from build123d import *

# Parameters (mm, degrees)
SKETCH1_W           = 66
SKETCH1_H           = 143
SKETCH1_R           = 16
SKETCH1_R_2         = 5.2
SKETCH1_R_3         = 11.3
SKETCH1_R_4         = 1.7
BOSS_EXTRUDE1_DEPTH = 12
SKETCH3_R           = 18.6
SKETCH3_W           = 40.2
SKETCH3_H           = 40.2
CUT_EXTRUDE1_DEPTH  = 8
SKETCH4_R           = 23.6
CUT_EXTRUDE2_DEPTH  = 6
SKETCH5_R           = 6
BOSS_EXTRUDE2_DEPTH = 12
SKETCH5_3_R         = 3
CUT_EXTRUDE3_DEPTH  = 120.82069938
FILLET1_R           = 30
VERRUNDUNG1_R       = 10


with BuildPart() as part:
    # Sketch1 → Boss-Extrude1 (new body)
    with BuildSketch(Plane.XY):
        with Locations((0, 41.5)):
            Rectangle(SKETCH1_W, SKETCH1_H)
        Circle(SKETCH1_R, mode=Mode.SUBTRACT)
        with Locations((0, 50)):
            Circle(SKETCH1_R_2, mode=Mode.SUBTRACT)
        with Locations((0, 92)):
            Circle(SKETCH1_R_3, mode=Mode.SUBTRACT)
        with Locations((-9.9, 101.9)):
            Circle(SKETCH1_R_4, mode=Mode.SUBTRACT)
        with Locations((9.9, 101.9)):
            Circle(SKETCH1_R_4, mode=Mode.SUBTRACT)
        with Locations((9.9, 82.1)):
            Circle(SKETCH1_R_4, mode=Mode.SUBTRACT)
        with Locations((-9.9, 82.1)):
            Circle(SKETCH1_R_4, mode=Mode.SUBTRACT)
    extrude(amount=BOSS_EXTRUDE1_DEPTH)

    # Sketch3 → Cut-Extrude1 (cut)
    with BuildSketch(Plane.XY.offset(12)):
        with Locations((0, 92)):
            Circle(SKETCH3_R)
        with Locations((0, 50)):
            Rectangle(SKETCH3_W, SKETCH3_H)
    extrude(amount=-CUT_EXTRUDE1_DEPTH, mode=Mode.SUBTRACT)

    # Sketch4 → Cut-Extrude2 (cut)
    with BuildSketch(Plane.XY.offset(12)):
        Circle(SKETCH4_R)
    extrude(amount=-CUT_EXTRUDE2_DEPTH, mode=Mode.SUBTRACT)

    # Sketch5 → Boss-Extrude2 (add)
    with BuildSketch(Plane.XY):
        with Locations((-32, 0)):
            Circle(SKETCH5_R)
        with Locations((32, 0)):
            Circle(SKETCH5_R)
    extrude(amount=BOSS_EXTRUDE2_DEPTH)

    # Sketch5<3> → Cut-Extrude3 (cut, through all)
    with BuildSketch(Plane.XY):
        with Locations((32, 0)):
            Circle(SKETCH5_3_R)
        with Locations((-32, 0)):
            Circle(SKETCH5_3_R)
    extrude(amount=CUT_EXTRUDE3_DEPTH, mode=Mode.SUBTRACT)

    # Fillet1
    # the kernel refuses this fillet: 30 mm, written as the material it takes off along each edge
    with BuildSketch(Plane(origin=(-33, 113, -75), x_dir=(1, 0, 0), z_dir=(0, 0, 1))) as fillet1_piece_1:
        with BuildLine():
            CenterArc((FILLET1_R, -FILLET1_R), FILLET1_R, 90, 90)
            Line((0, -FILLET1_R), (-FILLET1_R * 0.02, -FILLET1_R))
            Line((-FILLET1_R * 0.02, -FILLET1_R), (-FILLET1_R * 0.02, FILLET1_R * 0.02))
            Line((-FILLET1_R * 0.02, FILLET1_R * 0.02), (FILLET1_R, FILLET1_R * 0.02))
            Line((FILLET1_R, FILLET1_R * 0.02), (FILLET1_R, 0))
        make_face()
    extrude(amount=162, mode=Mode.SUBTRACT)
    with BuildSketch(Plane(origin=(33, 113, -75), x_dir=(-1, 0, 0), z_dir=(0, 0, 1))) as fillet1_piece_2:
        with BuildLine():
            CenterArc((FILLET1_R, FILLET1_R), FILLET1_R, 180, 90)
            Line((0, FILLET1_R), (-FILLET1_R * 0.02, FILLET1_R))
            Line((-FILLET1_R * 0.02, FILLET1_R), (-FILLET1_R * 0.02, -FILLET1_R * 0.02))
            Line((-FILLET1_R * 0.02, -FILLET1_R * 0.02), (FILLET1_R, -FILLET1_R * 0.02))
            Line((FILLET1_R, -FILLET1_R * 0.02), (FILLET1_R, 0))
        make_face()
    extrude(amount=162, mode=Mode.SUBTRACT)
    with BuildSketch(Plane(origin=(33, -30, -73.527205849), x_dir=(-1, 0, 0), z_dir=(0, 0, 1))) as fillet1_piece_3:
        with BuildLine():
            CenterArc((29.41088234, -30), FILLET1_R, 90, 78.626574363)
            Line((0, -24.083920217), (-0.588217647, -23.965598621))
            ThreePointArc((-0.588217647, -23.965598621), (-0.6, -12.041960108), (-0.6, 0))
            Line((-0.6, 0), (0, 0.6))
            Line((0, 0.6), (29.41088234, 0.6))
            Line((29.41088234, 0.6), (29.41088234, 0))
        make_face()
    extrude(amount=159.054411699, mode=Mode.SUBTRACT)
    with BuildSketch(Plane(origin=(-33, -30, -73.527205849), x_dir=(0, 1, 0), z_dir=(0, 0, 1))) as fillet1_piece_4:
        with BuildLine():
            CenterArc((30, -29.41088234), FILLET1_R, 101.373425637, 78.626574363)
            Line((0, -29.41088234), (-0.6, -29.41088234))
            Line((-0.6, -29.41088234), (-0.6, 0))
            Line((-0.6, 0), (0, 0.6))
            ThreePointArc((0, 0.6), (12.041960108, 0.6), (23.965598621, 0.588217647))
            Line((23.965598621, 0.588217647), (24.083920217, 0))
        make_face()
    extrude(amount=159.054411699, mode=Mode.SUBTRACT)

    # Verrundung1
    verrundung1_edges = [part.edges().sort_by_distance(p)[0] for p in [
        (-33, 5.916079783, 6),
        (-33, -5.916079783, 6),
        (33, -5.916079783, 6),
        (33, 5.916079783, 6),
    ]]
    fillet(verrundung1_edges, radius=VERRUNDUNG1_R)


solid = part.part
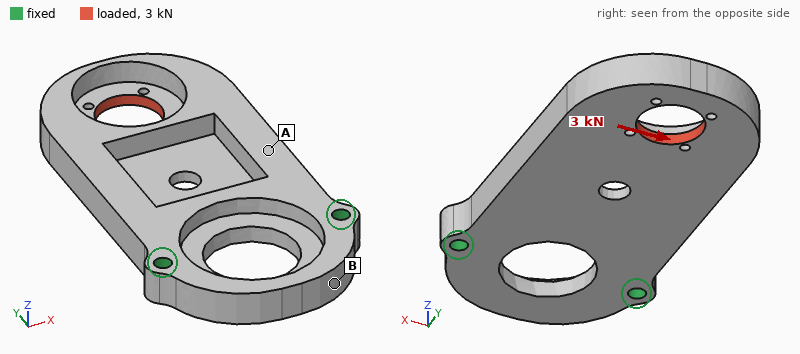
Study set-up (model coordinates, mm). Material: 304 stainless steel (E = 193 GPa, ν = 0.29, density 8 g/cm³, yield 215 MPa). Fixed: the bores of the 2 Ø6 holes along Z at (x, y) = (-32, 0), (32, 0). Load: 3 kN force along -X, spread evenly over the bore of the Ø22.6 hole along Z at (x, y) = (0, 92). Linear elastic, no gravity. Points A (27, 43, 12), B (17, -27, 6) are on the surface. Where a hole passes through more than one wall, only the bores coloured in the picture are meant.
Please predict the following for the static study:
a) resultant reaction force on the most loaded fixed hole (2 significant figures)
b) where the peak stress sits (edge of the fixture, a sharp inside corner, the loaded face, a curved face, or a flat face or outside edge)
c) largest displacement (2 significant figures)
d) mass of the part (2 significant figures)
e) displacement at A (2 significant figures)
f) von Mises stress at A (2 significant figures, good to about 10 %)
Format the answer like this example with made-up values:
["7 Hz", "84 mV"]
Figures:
["4.6 kN", "a curved face", "44 µm", "530 g", "11 µm", "15 MPa"]
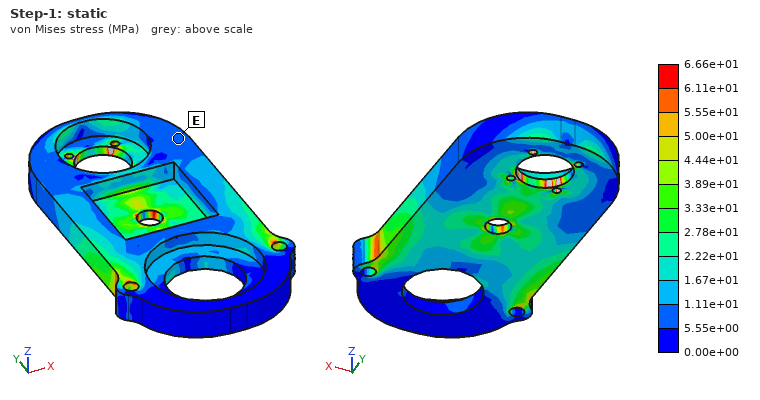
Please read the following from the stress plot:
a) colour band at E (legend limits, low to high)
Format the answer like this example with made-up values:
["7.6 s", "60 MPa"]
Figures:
["5.55e+00 to 1.11e+01 MPa"]
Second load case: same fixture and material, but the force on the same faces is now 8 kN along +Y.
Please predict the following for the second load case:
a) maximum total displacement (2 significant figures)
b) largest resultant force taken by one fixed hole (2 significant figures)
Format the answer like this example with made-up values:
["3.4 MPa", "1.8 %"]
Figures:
["0.16 mm", "4.1 kN"]
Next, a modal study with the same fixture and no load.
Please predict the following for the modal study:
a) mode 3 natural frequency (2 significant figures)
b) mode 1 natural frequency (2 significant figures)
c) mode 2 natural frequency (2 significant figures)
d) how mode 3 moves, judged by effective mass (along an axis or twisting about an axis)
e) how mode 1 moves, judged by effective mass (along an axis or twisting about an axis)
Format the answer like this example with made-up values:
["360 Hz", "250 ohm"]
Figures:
["3800 Hz", "730 Hz", "2000 Hz", "along X", "along Z"]
